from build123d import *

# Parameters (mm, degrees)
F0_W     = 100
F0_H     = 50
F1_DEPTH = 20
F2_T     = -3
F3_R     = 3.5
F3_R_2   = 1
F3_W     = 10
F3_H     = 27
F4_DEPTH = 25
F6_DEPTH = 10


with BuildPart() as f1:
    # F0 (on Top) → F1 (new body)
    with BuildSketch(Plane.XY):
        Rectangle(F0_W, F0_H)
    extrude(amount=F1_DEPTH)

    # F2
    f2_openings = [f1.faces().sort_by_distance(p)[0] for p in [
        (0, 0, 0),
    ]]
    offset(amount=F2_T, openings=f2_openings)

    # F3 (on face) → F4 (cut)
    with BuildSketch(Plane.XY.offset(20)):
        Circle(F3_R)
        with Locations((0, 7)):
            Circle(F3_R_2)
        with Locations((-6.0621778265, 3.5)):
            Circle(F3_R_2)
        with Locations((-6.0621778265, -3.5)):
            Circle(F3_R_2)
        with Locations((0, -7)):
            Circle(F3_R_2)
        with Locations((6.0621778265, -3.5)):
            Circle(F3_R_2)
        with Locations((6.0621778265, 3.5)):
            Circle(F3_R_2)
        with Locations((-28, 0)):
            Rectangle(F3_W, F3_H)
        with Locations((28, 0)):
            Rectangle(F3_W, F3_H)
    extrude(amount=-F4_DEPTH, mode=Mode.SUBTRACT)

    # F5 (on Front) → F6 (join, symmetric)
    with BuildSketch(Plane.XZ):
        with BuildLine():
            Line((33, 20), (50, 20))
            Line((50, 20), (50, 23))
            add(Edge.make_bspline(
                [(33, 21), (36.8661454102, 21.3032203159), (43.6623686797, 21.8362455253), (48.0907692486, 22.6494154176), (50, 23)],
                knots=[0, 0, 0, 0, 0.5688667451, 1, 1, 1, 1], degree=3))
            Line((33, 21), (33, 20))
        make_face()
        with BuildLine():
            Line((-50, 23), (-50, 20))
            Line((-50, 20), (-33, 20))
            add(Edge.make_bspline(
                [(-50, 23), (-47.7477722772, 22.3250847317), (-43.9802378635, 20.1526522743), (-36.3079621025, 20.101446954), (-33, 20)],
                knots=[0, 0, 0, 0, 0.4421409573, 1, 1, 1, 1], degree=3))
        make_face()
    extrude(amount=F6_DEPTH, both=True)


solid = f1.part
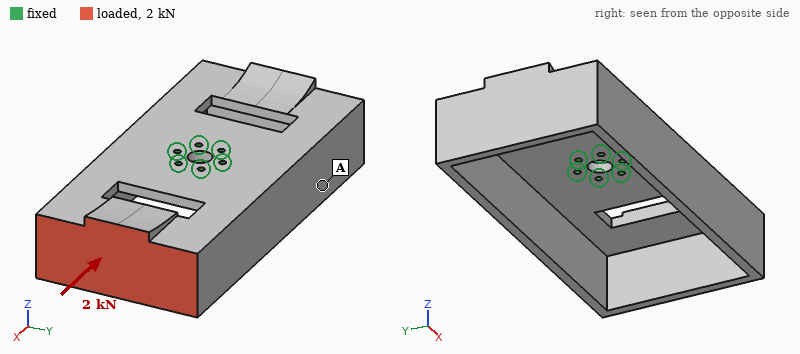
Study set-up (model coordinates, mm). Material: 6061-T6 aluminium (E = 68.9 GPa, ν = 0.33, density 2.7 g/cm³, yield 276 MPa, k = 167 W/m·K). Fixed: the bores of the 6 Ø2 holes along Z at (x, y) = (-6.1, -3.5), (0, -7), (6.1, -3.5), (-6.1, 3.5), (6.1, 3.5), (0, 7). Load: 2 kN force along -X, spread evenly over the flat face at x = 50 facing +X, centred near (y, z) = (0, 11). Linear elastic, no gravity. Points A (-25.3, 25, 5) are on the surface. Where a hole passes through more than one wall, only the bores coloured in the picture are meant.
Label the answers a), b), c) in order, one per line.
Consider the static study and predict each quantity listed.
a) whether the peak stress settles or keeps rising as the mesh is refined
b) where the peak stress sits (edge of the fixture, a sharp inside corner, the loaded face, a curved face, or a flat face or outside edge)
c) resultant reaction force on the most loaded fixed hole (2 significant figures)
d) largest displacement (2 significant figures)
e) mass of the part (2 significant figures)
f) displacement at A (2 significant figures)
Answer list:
a) keeps rising
b) edge of the fixture
c) 480 N
d) 0.46 mm
e) 78 g
f) 0.20 mm
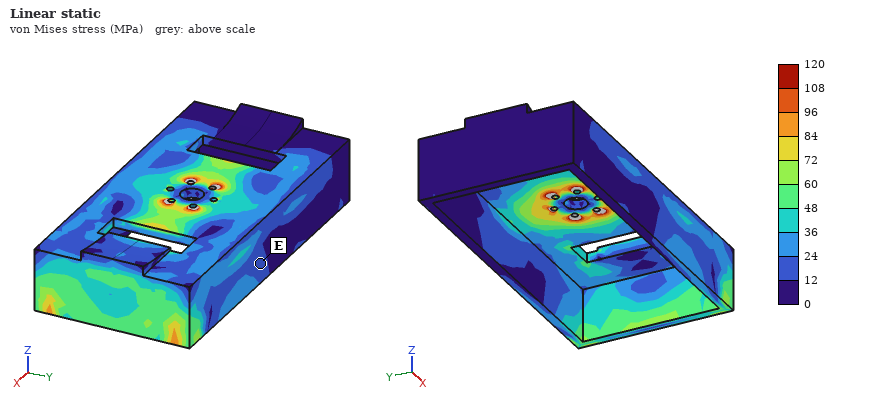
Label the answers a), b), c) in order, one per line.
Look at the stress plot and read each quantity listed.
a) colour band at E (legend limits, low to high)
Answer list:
a) 12 to 24 MPa
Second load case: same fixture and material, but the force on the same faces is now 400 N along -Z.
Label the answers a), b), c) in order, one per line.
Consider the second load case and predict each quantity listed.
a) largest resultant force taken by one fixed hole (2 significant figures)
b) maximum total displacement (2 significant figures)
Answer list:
a) 460 N
b) 0.54 mm
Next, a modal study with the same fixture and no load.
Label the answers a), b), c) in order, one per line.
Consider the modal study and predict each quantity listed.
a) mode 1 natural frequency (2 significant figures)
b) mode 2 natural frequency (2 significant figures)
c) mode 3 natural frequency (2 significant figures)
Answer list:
a) 800 Hz
b) 1500 Hz
c) 1600 Hz
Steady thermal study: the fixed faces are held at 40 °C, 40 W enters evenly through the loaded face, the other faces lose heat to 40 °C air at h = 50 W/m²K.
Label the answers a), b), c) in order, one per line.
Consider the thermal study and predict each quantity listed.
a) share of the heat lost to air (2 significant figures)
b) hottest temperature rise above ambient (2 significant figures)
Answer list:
a) 40 %
b) 59 K
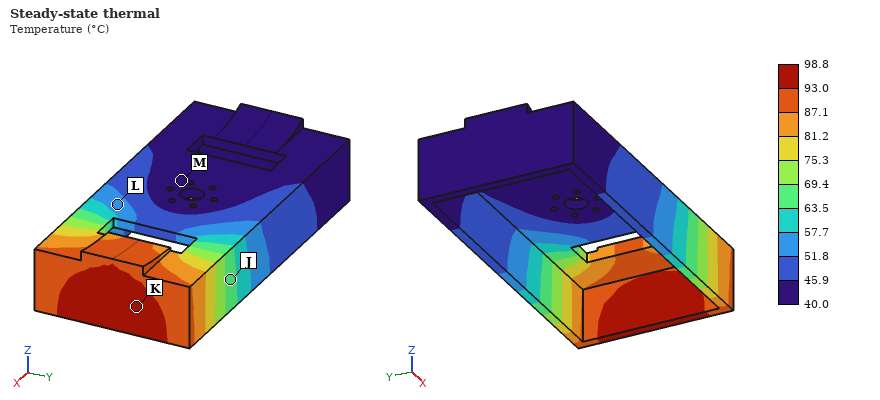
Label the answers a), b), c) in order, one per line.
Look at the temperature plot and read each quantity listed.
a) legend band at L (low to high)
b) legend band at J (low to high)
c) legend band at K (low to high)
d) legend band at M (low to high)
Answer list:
a) 51.8 to 57.7 °C
b) 63.5 to 69.4 °C
c) 93.0 to 98.8 °C
d) 40.0 to 45.9 °C
